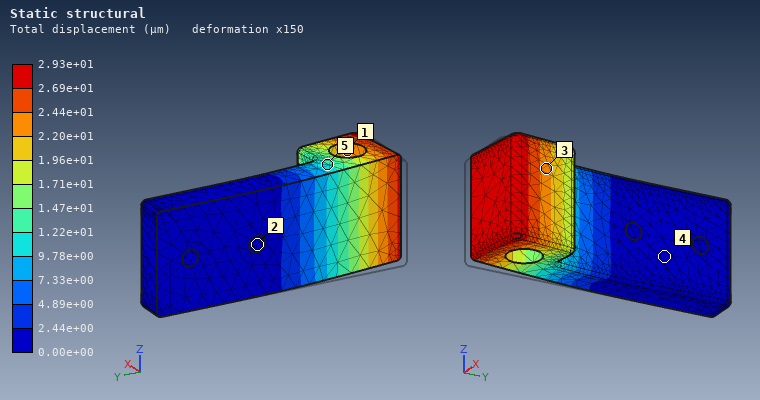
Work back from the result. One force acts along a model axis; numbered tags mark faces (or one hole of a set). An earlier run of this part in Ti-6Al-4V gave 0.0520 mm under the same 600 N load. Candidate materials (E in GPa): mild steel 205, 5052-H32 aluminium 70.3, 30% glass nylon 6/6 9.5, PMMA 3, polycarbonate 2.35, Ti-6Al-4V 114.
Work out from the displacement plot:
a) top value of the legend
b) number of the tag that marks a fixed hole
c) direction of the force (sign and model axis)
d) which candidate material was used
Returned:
2.93e+01 µm
2
+X
mild steel
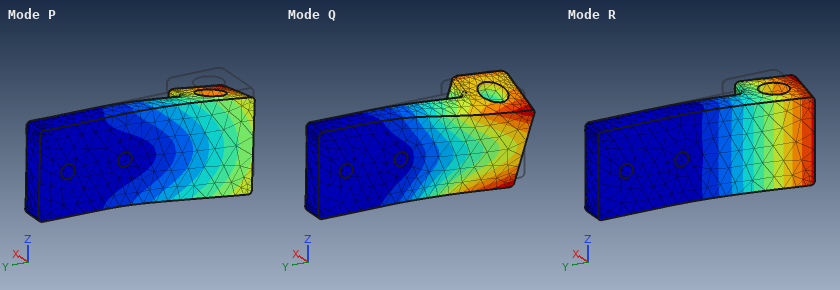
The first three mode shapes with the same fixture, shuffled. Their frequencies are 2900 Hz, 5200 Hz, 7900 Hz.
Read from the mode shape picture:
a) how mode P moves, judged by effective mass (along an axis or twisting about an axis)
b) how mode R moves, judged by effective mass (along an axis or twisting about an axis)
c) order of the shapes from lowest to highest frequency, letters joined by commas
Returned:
along Z
along X
R, P, Q
